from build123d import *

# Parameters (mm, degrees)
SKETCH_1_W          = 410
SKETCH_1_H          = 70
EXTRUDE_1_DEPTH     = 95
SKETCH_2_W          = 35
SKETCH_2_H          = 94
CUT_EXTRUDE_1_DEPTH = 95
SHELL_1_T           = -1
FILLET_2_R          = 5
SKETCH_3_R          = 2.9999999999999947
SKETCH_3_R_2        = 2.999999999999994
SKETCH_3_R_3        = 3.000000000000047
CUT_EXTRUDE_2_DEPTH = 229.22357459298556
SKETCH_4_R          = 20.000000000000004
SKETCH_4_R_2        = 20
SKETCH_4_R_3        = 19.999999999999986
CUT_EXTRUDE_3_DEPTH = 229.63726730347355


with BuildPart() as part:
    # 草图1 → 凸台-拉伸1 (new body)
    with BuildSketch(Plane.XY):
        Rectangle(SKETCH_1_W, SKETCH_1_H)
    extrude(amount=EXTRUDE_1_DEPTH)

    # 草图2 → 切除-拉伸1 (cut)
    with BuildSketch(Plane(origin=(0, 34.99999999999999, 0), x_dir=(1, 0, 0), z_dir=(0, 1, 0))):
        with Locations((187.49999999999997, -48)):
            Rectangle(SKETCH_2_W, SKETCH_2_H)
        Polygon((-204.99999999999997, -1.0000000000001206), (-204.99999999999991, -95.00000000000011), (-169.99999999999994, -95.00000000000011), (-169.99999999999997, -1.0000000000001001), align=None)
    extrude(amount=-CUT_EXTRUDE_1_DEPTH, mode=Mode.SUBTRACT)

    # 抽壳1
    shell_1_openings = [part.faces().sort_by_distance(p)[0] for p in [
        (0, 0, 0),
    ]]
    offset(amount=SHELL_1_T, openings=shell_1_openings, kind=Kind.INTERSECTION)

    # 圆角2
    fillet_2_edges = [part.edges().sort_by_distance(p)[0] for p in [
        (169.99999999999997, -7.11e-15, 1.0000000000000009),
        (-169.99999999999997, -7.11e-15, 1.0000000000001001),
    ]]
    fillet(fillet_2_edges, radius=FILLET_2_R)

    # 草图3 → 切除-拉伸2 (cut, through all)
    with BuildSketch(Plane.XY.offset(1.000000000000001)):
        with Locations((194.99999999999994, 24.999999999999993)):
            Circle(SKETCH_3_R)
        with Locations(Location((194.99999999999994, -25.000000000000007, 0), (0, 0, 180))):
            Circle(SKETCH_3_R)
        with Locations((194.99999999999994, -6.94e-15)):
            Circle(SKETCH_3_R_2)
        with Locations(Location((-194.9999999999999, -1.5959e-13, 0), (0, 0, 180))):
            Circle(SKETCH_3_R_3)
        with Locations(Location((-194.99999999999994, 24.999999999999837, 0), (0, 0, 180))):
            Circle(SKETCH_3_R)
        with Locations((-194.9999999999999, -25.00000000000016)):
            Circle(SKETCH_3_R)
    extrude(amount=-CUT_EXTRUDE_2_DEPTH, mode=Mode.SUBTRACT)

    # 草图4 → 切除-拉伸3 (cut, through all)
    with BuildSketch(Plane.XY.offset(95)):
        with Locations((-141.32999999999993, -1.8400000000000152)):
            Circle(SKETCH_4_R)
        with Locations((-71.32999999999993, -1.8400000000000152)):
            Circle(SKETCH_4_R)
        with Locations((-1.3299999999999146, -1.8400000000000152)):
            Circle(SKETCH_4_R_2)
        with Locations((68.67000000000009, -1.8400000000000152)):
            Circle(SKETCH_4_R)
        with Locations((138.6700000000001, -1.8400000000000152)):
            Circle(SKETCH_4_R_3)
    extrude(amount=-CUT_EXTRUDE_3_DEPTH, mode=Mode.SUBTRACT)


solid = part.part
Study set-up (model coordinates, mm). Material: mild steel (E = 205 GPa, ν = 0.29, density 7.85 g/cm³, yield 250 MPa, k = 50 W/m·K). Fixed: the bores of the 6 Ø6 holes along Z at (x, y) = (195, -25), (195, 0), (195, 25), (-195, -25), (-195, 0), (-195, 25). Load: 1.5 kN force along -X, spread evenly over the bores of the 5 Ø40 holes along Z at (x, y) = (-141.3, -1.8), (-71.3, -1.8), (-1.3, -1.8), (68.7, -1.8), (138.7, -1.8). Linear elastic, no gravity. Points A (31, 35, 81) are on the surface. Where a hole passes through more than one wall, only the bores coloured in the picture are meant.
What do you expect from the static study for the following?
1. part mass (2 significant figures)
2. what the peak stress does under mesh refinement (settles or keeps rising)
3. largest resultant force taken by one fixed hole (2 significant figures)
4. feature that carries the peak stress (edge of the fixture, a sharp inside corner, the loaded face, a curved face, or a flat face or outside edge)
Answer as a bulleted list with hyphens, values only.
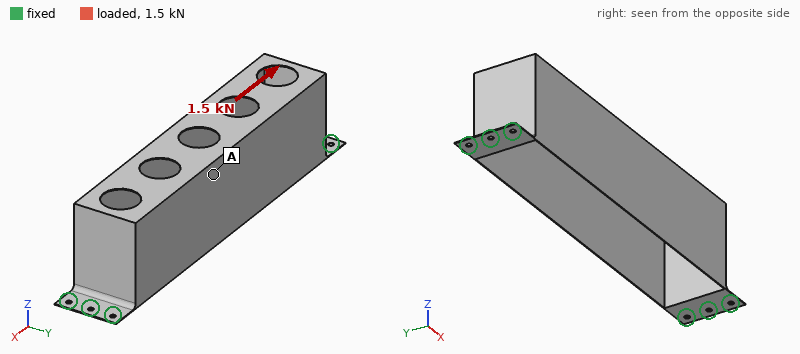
- 780 g
- keeps rising
- 340 N
- edge of the fixture
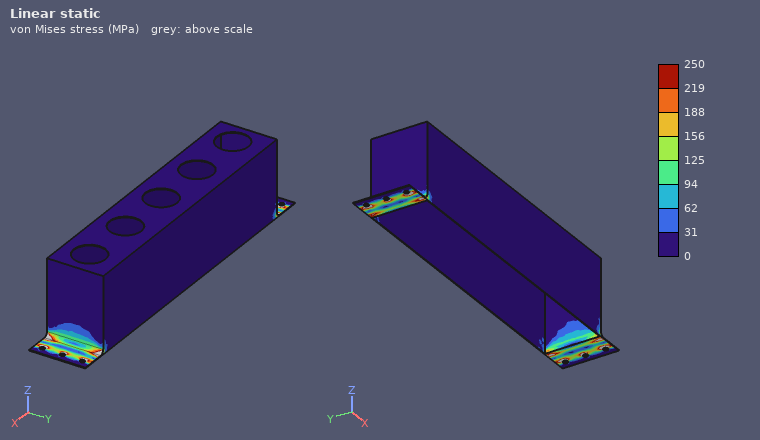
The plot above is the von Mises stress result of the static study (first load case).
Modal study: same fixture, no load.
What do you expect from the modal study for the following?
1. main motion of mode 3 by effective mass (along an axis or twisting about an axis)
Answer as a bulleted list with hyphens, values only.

- twisting about X
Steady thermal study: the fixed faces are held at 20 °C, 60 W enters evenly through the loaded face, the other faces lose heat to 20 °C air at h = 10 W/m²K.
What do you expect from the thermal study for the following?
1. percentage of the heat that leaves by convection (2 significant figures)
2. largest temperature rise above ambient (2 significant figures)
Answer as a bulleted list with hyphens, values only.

- 97 %
- 87 K
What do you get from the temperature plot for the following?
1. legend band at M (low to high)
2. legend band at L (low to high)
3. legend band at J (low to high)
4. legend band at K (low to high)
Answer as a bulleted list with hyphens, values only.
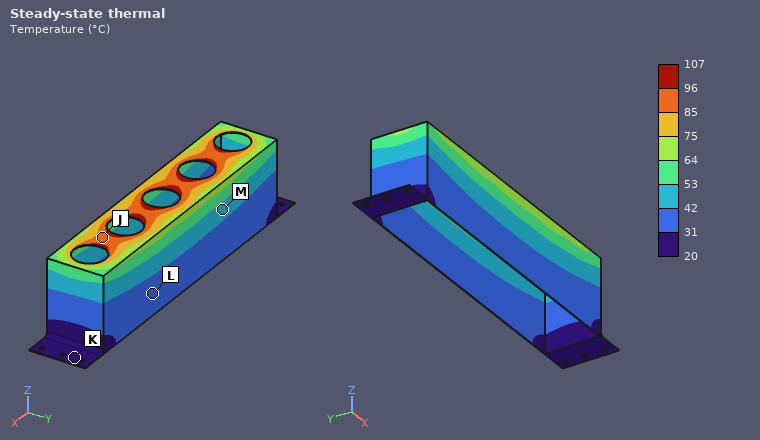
- 42 to 53 °C
- 31 to 42 °C
- 85 to 96 °C
- 20 to 31 °C
